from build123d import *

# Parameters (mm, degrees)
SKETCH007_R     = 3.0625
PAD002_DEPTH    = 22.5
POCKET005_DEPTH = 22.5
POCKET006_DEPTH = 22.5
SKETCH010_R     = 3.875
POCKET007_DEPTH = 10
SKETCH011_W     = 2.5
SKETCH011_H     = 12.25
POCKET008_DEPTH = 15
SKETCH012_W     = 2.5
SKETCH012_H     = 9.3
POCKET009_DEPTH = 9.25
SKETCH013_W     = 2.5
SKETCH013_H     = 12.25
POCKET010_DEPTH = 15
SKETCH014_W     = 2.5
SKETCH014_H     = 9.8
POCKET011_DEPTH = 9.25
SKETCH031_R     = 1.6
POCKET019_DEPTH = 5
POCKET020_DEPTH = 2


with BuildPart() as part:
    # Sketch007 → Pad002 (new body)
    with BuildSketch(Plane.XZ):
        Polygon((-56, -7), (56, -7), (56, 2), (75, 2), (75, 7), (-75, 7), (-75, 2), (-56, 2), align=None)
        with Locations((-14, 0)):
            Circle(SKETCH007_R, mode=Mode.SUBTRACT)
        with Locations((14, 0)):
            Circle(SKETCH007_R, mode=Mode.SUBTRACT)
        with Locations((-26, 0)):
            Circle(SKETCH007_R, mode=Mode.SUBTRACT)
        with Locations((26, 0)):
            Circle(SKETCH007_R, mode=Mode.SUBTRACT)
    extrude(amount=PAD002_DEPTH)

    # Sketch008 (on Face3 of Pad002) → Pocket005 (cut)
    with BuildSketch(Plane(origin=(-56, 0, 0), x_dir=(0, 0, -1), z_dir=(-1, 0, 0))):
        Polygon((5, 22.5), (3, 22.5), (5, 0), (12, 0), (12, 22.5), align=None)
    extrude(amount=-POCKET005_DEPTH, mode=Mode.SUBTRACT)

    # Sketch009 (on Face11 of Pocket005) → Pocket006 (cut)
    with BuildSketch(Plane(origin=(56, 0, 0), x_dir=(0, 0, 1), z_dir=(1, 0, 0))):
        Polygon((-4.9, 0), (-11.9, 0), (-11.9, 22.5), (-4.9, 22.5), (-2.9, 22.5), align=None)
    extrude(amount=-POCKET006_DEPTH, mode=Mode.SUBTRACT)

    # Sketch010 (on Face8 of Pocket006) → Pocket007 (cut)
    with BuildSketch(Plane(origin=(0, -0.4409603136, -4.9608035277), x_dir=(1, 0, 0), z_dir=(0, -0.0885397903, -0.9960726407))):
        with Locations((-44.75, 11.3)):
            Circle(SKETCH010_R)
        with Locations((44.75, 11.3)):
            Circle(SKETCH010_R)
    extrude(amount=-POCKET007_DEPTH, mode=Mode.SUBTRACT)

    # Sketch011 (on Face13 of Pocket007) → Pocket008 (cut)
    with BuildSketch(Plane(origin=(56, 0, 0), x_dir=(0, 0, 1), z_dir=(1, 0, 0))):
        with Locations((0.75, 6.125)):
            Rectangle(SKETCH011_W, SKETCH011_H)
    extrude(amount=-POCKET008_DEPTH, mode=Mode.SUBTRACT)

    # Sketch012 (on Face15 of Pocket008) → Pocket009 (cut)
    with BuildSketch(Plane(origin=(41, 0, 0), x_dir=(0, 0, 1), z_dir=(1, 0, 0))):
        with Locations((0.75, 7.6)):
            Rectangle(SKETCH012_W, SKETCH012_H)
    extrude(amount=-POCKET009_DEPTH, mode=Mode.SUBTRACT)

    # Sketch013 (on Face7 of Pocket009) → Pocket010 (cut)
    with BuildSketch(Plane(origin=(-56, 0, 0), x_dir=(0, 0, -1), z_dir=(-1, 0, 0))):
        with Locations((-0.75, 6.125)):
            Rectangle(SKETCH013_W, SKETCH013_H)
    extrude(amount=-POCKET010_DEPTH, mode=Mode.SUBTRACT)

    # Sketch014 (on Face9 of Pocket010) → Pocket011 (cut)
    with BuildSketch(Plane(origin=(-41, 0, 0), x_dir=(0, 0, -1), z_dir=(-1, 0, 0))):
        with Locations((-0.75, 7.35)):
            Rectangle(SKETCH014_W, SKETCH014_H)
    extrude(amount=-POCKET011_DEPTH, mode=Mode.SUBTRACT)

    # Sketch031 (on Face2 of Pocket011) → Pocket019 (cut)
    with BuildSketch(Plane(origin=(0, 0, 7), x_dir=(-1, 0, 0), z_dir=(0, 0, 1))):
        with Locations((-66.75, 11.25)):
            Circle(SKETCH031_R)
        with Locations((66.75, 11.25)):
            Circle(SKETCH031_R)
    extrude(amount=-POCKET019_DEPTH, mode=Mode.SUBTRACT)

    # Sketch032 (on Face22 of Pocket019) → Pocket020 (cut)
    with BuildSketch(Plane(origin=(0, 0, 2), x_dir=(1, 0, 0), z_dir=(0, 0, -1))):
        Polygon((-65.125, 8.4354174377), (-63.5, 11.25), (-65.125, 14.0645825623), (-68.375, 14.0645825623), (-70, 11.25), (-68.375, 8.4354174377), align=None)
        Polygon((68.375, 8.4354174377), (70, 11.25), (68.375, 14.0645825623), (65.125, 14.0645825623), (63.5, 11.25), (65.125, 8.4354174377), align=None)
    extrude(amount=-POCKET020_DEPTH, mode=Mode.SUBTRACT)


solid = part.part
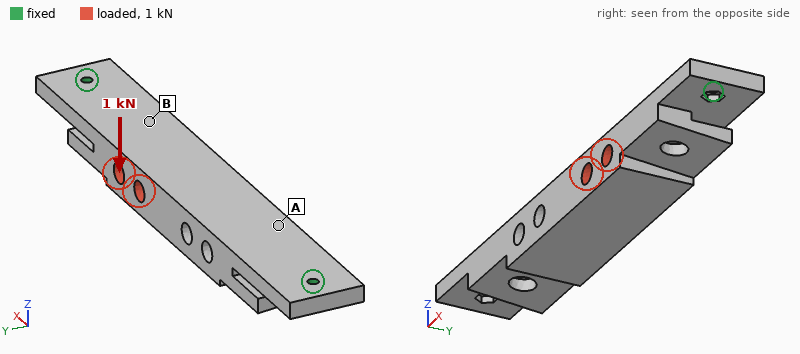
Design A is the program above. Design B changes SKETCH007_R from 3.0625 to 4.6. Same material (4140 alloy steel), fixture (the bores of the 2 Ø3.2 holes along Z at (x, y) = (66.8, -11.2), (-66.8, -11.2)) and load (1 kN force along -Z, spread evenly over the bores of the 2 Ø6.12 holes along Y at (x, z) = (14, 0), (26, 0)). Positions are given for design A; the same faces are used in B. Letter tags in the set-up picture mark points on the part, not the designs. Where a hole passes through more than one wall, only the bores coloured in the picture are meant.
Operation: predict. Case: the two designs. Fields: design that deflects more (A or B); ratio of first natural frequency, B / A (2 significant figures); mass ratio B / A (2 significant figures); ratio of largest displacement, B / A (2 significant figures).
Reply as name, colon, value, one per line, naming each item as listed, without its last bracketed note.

design that deflects more: B
ratio of first natural frequency, B / A: 1.0
mass ratio B / A: 0.89
ratio of largest displacement, B / A: 1.1
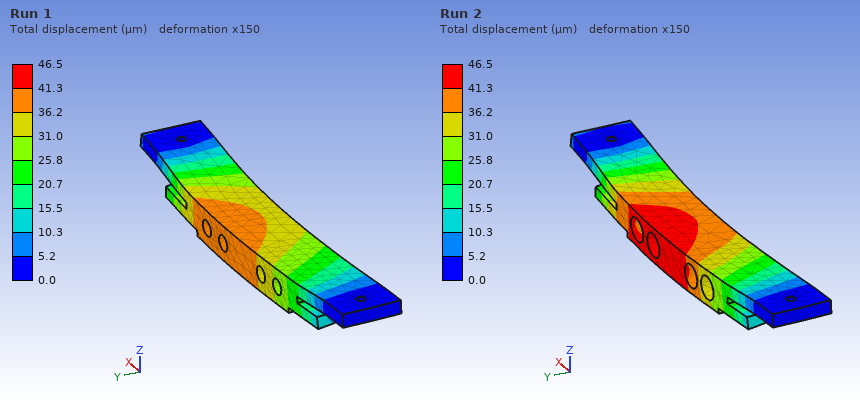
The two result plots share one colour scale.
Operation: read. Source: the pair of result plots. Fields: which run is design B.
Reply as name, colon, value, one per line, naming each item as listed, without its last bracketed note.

which run is design B: Run 2
